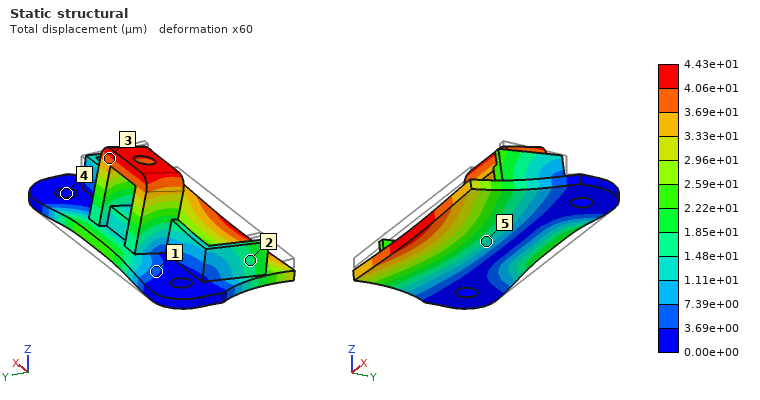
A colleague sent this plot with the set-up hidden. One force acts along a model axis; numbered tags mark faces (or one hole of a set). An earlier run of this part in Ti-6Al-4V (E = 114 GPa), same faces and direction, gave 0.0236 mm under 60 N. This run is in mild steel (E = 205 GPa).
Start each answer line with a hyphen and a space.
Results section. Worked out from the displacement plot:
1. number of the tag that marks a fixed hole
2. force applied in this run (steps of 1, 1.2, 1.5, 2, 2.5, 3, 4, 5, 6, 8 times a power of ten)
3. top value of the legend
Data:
- 4
- 200 N
- 4.43e+01 µm
